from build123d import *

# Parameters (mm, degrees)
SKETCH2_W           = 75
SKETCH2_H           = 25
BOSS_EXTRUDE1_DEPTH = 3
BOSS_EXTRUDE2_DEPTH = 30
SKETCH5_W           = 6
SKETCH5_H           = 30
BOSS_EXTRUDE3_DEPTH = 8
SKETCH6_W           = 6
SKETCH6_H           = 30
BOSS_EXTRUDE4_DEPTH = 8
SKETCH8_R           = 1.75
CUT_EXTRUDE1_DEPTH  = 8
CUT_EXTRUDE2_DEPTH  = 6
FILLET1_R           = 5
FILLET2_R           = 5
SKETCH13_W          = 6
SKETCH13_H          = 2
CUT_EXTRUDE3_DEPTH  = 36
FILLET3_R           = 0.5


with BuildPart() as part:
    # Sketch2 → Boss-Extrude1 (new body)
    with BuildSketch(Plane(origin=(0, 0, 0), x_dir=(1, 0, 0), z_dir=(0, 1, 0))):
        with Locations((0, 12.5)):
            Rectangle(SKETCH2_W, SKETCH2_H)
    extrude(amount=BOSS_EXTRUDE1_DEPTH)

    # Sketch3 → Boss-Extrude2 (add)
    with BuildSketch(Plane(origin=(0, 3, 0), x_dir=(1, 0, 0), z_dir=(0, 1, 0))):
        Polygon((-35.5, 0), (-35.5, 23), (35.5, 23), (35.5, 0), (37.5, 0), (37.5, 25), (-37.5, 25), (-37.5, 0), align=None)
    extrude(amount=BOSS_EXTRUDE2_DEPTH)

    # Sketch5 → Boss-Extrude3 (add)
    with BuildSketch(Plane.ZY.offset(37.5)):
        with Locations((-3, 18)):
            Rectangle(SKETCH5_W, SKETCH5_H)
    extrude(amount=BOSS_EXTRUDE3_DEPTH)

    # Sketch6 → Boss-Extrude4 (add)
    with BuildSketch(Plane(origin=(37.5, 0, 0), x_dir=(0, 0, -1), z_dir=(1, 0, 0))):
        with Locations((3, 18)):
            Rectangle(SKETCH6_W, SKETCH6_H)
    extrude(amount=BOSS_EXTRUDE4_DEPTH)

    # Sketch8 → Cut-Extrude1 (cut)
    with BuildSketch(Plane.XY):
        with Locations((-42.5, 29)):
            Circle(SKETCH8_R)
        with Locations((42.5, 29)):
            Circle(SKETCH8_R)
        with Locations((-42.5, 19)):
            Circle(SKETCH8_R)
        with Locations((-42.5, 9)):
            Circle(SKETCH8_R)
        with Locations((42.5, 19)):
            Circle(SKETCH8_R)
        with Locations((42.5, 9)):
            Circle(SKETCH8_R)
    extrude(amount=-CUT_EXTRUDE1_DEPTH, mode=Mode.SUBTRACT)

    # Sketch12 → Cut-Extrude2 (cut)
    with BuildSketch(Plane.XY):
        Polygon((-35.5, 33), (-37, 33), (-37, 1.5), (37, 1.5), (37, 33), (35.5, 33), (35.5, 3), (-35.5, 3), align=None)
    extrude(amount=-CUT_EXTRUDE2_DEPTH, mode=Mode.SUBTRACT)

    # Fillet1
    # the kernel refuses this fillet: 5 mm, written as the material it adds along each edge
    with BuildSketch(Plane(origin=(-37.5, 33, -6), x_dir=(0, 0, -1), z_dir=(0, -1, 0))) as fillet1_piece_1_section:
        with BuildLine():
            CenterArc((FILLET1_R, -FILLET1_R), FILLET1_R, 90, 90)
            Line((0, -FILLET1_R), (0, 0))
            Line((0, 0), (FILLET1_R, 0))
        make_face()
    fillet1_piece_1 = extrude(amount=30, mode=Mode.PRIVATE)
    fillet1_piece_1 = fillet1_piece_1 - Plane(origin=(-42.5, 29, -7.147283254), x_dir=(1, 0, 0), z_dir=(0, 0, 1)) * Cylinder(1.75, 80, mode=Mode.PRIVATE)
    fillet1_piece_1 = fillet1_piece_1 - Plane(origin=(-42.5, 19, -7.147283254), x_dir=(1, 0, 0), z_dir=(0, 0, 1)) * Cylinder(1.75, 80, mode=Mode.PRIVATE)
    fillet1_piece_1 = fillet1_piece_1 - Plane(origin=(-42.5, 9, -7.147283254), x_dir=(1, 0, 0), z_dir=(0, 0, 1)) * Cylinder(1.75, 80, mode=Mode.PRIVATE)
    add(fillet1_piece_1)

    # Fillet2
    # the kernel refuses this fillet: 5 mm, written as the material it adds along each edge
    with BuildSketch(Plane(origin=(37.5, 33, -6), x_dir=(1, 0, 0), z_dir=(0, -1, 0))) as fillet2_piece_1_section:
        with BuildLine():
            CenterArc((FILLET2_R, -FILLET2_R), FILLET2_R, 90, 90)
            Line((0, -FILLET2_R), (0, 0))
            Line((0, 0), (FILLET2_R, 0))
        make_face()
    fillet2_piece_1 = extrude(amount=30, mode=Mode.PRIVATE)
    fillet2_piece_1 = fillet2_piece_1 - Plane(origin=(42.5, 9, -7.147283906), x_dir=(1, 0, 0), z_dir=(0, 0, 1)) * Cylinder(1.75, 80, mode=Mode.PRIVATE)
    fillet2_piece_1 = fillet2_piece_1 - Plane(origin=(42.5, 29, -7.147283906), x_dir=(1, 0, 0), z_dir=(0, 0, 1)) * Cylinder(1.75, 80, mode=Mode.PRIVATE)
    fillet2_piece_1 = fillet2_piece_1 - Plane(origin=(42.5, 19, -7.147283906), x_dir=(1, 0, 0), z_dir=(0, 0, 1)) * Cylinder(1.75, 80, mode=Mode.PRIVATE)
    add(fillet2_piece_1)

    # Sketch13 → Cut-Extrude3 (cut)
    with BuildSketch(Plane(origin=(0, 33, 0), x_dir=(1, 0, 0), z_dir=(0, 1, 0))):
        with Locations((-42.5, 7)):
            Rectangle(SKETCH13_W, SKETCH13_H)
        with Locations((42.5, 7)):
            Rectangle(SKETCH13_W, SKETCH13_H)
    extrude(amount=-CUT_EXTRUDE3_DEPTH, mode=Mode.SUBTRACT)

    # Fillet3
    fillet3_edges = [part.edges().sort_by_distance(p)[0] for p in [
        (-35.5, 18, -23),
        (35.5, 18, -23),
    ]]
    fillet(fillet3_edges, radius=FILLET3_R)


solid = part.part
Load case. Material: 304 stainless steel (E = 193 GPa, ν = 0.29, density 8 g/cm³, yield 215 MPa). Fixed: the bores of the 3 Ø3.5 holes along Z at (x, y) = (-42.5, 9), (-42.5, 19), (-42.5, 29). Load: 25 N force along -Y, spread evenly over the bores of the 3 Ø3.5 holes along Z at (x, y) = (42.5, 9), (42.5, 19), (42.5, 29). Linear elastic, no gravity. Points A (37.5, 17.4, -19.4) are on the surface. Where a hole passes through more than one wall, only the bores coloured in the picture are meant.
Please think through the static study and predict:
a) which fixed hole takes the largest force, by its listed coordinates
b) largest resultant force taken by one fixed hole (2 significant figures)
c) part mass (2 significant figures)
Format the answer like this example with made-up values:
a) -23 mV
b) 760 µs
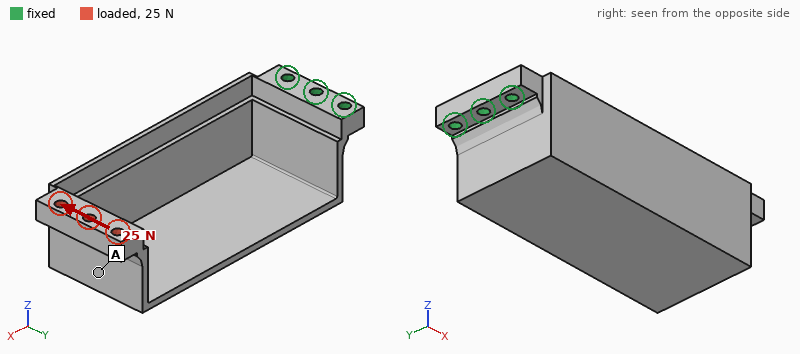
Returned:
a) (-42.5, 9)
b) 120 N
c) 120 g
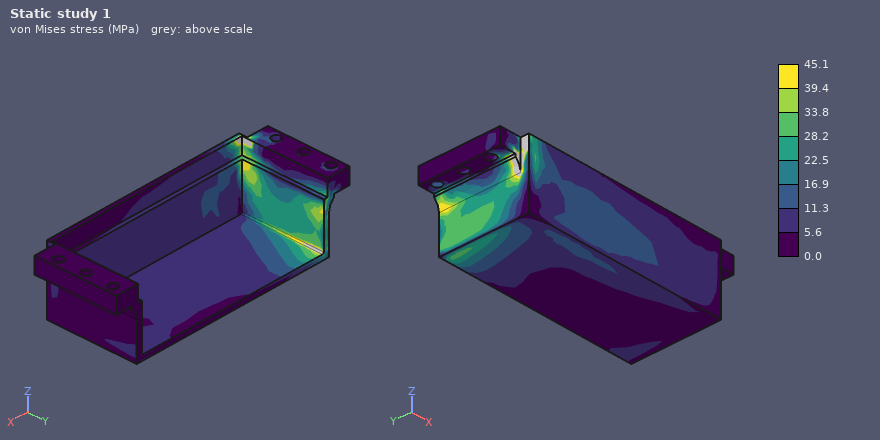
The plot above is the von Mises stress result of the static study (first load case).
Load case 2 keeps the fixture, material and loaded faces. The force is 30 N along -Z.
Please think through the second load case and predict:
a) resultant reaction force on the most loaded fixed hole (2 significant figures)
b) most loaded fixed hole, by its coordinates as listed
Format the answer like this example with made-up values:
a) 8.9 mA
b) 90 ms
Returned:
a) 60 N
b) (-42.5, 19)
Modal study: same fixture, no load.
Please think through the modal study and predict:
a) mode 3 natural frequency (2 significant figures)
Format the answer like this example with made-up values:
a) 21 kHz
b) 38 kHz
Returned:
a) 1100 Hz
